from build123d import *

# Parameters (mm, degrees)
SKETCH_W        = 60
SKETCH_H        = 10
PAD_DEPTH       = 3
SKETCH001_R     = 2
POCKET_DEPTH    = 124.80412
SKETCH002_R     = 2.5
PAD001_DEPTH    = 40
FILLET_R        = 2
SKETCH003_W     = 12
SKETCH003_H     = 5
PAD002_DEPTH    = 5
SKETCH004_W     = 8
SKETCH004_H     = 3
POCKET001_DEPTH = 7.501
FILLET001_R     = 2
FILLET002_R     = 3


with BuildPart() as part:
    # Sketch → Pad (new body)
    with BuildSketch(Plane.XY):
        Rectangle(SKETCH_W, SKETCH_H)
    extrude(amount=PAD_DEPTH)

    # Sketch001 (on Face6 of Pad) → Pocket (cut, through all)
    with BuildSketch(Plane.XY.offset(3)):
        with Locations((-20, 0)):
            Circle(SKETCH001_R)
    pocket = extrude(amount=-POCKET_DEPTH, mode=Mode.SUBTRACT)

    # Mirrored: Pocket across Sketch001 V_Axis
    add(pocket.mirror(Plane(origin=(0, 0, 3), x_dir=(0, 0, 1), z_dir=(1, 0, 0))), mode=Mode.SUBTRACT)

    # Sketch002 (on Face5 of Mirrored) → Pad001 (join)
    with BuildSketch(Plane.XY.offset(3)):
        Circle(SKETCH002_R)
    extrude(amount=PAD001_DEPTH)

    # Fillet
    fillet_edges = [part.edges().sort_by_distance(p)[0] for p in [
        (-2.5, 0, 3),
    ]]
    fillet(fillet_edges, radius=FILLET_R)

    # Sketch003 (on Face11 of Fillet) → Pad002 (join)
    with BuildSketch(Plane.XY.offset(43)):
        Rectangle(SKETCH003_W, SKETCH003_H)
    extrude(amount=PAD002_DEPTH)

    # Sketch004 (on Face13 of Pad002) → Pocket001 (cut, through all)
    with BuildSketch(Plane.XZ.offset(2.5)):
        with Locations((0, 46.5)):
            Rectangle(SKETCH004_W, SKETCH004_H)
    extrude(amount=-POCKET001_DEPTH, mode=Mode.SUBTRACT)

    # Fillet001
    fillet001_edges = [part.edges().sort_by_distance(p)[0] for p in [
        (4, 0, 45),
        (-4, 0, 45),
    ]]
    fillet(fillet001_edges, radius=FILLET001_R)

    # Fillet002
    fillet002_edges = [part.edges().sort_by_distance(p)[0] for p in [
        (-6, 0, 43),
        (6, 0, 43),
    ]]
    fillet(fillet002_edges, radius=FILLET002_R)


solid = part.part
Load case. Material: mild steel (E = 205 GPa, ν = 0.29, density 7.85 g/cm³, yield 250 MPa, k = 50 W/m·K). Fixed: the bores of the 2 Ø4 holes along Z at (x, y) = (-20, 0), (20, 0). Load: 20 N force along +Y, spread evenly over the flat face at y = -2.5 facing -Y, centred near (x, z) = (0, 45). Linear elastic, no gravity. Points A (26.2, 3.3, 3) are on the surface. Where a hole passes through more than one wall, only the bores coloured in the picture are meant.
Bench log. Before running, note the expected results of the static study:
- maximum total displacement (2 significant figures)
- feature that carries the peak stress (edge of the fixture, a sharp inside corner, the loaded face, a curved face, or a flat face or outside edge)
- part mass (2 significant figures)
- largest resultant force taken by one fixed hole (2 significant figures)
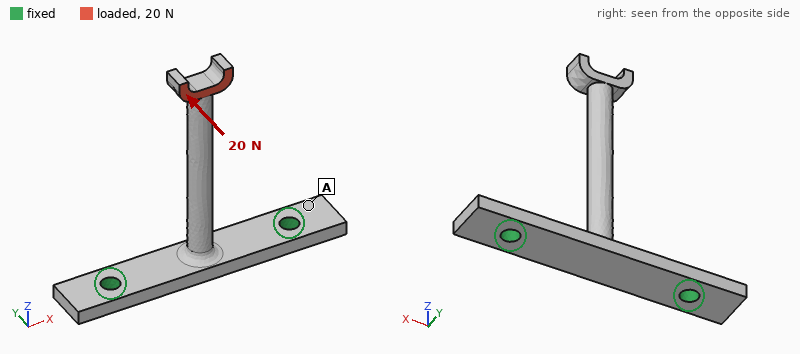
0.14 mm
a curved face
21 g
10 N
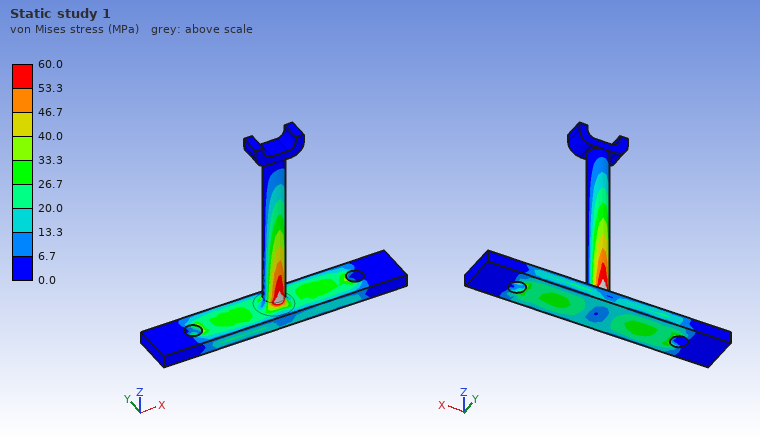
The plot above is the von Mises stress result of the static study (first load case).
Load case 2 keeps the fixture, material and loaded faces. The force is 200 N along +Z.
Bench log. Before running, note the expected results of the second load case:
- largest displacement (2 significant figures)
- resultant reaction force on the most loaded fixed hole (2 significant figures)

0.11 mm
100 N
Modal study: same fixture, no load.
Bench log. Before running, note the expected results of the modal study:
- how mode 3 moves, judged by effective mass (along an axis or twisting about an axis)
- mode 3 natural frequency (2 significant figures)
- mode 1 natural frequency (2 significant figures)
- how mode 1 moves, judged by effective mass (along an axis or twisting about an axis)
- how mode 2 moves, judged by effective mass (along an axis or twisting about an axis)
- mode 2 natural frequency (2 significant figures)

along Z
6500 Hz
1200 Hz
along Y
along X
1400 Hz
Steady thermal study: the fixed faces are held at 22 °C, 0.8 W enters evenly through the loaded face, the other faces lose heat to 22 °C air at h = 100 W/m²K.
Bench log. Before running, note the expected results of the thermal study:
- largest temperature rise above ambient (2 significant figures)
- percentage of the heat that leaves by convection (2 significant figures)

15 K
83 %
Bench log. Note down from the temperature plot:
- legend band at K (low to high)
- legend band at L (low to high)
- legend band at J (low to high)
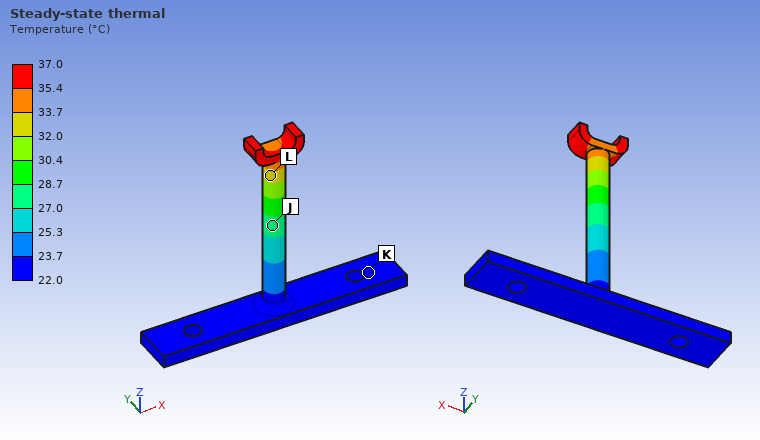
22.0 to 23.7 °C
32.0 to 33.7 °C
27.0 to 28.7 °C
